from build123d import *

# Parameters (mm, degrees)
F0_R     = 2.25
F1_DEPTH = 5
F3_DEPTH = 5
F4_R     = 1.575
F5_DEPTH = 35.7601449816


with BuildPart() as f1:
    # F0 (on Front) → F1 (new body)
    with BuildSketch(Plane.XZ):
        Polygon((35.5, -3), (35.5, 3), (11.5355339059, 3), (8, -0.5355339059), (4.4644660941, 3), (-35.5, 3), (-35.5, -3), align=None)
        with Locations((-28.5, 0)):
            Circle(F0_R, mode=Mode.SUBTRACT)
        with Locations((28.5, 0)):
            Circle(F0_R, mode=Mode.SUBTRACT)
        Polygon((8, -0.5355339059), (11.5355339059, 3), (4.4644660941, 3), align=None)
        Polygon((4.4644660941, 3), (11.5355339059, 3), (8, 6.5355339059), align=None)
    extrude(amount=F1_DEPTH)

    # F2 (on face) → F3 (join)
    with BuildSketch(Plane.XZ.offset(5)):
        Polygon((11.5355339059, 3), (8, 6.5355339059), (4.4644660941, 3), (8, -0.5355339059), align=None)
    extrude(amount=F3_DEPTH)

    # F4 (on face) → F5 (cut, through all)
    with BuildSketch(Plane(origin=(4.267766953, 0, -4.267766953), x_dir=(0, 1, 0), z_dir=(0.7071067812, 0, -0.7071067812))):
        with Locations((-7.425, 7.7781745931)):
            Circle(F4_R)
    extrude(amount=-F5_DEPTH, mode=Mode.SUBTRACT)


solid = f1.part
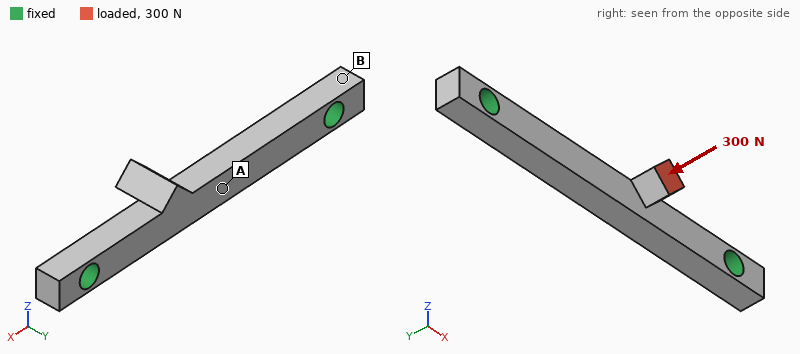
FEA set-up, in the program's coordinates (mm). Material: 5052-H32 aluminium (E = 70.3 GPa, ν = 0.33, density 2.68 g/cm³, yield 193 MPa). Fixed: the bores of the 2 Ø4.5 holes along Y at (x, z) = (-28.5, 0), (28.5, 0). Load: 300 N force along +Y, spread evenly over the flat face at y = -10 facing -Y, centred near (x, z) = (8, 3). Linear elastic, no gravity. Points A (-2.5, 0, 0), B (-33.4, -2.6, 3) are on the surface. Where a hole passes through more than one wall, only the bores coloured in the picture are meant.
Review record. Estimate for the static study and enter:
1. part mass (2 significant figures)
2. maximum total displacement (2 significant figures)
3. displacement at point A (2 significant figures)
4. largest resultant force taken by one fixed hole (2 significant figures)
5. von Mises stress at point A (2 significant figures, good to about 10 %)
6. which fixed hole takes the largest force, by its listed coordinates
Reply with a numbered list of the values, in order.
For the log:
1. 5.7 g
2. 71 µm
3. 42 µm
4. 210 N
5. 36 MPa
6. (28.5, 0)
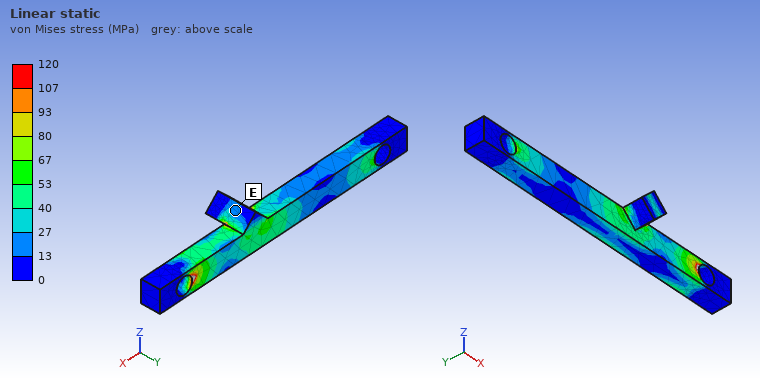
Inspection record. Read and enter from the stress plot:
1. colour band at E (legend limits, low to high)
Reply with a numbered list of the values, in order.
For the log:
1. 13 to 27 MPa
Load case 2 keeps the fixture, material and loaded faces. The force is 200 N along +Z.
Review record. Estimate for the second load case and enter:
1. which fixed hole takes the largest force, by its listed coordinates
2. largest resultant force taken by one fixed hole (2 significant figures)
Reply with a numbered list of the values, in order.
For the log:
1. (28.5, 0)
2. 140 N
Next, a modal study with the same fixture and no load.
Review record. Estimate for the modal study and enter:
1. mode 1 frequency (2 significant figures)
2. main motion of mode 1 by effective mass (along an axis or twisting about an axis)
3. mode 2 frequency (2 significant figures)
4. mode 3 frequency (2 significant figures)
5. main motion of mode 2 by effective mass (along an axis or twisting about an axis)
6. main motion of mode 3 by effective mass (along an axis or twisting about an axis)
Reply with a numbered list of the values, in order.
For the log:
1. 8100 Hz
2. along Y
3. 9200 Hz
4. 18 kHz
5. along Z
6. twisting about X
